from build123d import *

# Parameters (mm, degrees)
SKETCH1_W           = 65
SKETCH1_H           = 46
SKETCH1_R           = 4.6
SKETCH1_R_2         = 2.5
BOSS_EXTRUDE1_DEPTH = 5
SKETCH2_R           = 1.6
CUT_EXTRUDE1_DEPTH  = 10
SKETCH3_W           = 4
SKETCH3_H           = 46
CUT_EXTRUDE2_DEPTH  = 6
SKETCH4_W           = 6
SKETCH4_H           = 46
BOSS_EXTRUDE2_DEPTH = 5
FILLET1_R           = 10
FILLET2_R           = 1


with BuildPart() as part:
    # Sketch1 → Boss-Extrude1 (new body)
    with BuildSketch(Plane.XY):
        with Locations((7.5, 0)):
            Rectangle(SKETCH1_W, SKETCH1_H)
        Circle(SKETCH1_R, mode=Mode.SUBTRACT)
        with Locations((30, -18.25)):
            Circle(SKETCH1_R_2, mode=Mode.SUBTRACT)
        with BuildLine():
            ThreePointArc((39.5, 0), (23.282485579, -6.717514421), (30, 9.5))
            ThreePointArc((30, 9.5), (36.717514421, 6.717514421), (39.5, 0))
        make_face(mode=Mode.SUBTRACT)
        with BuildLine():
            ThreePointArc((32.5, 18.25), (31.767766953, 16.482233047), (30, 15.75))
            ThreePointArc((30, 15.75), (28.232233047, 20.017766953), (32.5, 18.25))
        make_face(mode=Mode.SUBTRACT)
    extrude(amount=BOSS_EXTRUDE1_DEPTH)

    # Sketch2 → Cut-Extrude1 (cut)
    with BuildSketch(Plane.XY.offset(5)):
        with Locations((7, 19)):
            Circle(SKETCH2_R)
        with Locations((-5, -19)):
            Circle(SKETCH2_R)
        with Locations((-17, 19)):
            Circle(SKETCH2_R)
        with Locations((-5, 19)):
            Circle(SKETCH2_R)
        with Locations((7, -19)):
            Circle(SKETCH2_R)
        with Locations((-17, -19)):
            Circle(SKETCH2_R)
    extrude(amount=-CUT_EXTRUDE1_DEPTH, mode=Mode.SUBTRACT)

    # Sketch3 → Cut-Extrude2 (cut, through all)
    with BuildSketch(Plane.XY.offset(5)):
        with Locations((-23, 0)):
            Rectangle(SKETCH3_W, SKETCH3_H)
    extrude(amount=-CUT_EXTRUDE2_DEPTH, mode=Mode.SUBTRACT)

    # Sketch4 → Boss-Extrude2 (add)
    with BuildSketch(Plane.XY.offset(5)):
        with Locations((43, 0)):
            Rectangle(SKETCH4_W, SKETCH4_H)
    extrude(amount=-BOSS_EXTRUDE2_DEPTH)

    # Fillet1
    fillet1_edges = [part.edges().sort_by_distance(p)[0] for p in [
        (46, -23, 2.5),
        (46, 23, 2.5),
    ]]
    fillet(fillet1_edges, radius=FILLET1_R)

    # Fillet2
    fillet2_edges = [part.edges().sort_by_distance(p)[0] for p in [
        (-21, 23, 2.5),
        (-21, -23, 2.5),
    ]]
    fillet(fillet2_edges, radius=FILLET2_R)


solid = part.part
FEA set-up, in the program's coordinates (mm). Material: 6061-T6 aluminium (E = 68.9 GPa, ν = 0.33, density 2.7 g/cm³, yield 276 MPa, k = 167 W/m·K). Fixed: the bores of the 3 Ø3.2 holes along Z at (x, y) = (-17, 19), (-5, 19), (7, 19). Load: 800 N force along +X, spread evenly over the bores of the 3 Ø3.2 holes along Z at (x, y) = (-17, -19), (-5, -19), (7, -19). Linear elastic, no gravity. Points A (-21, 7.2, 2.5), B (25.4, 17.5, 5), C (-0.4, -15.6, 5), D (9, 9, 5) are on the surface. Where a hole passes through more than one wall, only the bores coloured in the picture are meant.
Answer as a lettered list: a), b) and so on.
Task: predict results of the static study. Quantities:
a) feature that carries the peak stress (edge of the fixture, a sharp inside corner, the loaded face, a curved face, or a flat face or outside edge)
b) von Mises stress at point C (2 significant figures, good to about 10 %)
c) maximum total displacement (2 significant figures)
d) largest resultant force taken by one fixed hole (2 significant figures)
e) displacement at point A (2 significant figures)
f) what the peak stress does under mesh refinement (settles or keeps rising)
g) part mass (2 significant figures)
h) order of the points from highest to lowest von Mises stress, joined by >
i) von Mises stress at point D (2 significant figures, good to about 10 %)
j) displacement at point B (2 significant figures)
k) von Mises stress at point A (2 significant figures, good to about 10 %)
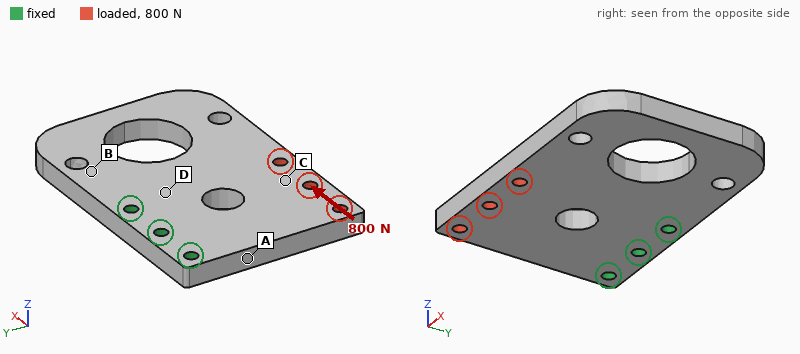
a) edge of the fixture
b) 11 MPa
c) 33 µm
d) 1.2 kN
e) 7.7 µm
f) keeps rising
g) 35 g
h) A > D > C > B
i) 15 MPa
j) 13 µm
k) 23 MPa
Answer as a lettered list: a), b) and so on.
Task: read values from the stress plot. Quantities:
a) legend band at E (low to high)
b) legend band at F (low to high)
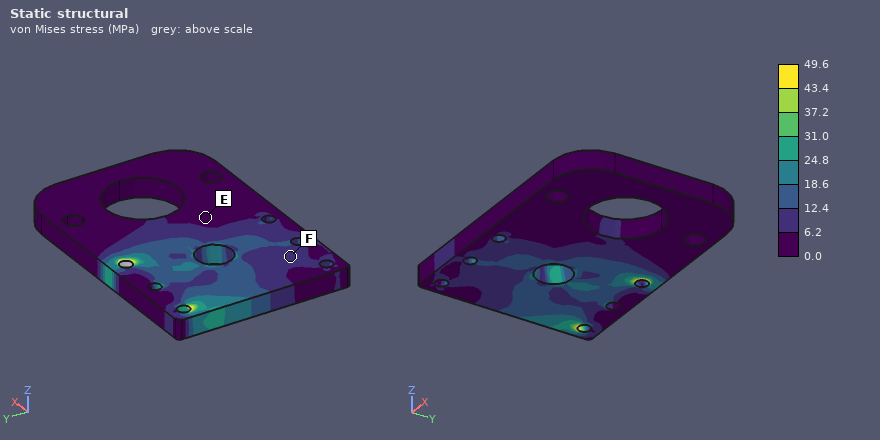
a) 0.0 to 6.2 MPa
b) 6.2 to 12.4 MPa
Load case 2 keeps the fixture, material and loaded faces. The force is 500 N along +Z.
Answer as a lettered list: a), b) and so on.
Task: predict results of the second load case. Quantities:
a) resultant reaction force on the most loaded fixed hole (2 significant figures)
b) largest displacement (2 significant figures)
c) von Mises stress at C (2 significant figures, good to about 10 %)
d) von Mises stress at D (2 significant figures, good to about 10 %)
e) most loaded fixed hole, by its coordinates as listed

a) 290 N
b) 0.39 mm
c) 19 MPa
d) 65 MPa
e) (-5, 19)
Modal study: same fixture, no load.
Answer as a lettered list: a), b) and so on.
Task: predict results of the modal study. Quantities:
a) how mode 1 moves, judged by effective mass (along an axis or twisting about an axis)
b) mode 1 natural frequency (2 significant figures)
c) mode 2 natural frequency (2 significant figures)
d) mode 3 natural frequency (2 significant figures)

a) along Z
b) 1600 Hz
c) 2500 Hz
d) 4700 Hz
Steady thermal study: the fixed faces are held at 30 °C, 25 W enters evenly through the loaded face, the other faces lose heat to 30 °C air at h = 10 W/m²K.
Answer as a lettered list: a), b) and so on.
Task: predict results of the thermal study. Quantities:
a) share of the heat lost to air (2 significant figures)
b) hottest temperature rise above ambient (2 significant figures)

a) 3.9 %
b) 34 K
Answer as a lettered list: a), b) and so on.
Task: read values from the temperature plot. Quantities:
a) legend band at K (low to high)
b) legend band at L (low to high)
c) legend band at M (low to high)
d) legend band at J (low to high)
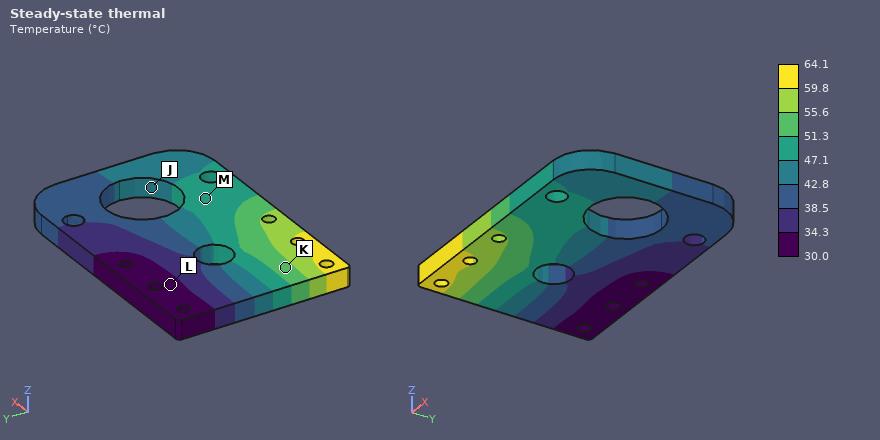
a) 51.3 to 55.6 °C
b) 30.0 to 34.3 °C
c) 47.1 to 51.3 °C
d) 42.8 to 47.1 °C
